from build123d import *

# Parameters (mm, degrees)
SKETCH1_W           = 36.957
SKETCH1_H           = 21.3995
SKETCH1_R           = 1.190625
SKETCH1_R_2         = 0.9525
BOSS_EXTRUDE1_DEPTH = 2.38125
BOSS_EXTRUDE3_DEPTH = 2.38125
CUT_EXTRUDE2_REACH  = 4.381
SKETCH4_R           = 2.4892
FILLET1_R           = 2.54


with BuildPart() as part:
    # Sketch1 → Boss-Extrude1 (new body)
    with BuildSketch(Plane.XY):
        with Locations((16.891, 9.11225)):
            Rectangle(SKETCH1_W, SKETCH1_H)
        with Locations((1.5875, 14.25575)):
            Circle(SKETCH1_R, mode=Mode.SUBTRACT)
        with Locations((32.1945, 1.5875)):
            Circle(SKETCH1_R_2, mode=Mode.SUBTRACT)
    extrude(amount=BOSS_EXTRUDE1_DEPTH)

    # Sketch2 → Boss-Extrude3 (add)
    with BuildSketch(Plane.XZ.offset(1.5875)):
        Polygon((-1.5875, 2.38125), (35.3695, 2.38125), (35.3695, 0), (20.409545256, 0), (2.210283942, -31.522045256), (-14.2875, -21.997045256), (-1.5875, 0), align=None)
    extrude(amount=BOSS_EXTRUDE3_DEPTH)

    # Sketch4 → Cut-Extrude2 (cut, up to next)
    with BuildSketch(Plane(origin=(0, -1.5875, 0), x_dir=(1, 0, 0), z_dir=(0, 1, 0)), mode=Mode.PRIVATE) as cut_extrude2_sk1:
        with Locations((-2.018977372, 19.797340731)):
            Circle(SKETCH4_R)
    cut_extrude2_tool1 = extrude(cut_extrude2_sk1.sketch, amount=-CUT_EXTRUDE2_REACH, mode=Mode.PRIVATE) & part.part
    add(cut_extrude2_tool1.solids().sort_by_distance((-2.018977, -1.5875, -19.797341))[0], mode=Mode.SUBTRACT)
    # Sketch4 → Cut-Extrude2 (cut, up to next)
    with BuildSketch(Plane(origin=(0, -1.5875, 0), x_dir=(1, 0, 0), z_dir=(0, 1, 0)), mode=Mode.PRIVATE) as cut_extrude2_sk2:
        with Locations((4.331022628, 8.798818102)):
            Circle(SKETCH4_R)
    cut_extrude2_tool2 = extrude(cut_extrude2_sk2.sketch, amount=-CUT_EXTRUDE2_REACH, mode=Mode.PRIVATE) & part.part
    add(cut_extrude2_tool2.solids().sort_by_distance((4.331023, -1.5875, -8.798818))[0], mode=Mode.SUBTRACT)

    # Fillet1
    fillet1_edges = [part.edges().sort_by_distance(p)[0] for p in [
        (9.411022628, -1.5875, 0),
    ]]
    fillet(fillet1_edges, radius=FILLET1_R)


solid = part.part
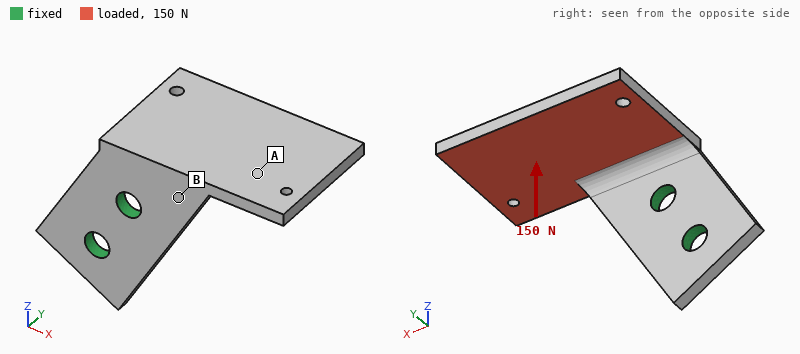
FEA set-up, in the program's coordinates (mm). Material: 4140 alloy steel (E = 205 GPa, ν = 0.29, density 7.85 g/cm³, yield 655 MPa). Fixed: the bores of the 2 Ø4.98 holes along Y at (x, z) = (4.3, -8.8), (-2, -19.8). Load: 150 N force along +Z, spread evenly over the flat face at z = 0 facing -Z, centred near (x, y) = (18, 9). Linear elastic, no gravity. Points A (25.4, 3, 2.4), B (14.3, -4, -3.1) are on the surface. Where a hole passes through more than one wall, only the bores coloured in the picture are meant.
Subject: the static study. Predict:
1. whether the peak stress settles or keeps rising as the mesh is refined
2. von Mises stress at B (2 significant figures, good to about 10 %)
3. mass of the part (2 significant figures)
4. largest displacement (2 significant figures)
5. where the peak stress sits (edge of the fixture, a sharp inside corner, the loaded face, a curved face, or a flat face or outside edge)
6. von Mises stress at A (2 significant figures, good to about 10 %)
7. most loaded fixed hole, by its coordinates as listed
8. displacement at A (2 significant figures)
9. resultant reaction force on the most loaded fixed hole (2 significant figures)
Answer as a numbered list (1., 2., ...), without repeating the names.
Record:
1. keeps rising
2. 78 MPa
3. 27 g
4. 0.14 mm
5. edge of the fixture
6. 16 MPa
7. (4.3, -8.8)
8. 0.049 mm
9. 190 N
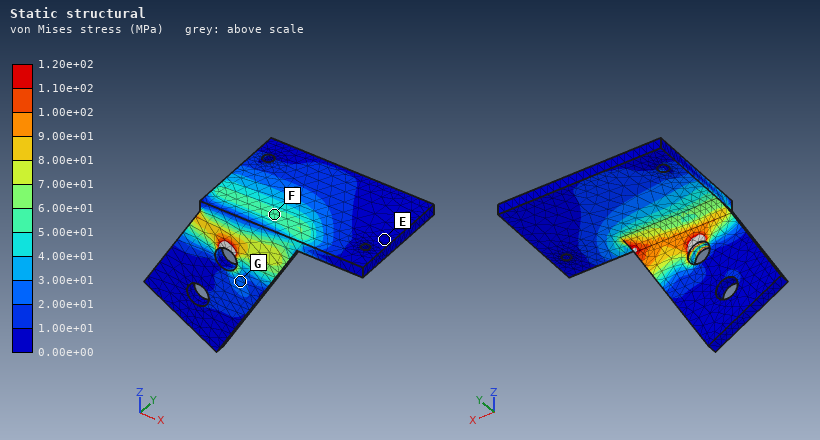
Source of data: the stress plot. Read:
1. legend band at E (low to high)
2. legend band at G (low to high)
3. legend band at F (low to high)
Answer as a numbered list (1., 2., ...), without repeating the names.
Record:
1. 0.00e+00 to 1.00e+01 MPa
2. 2.00e+01 to 3.00e+01 MPa
3. 5.00e+01 to 6.00e+01 MPa
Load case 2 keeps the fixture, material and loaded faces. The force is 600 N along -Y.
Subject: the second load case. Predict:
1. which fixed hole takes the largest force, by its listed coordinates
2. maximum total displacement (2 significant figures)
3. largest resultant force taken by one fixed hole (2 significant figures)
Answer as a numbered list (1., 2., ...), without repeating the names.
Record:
1. (4.3, -8.8)
2. 0.32 mm
3. 690 N
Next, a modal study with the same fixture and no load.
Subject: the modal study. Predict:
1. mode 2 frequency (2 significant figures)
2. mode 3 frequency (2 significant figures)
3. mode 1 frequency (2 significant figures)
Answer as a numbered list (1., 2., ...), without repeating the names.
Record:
1. 2400 Hz
2. 4100 Hz
3. 1600 Hz
